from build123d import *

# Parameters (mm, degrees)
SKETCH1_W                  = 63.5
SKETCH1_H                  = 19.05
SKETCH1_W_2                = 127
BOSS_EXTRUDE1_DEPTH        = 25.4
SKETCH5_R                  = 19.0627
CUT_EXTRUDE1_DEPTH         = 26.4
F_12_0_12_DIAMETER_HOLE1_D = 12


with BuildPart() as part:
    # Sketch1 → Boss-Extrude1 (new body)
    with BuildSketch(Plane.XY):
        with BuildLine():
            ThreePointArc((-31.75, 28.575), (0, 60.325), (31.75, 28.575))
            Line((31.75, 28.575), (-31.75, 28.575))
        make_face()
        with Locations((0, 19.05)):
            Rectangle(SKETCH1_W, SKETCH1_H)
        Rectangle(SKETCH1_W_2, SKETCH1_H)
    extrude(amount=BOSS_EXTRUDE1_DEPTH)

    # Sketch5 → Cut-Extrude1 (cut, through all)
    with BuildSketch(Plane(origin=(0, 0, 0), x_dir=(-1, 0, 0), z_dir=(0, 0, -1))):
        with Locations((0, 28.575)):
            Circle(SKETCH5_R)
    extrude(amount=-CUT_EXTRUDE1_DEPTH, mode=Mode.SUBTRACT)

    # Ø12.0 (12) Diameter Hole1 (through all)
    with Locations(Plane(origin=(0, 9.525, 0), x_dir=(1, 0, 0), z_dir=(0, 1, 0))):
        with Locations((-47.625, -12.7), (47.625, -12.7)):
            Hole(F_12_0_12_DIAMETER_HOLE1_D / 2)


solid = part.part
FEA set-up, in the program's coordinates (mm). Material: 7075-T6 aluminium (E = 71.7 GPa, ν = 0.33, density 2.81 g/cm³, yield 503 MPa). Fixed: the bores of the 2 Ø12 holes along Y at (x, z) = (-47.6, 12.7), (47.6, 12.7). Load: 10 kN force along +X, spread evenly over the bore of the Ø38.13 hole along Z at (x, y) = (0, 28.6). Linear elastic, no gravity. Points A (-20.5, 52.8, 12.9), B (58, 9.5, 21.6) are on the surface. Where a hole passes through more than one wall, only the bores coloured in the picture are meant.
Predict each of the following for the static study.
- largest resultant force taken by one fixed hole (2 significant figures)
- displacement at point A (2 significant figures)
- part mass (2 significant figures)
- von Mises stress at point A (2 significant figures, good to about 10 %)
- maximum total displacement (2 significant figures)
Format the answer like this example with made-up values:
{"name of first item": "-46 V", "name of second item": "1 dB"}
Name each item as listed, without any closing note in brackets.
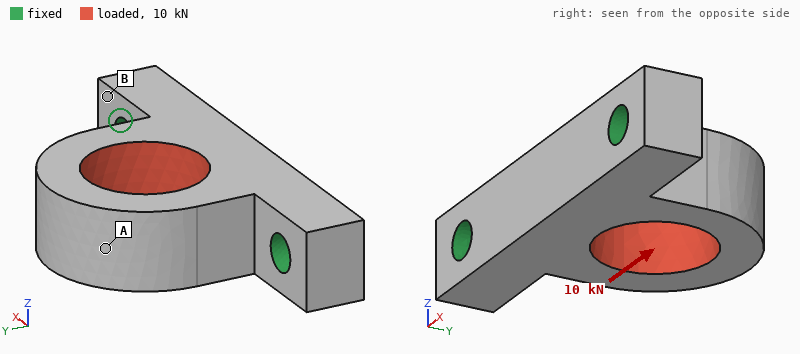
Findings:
{"largest resultant force taken by one fixed hole": "6.2 kN", "displacement at point A": "53 µm", "part mass": "280 g", "von Mises stress at point A": "20 MPa", "maximum total displacement": "54 µm"}
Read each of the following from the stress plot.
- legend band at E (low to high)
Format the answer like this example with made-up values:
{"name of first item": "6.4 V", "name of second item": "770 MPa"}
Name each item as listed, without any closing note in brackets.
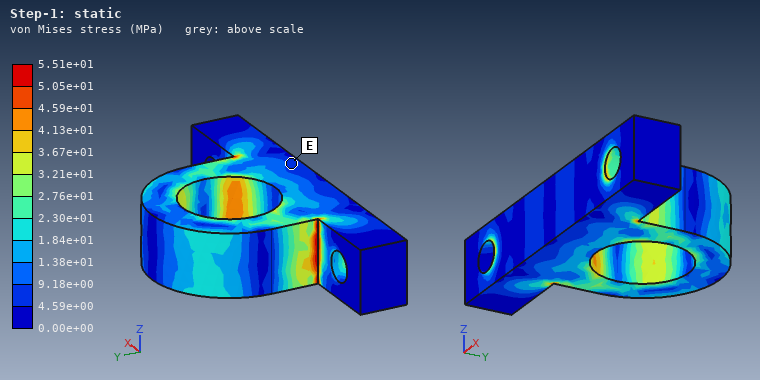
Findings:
{"legend band at E": "4.59e+00 to 9.18e+00 MPa"}
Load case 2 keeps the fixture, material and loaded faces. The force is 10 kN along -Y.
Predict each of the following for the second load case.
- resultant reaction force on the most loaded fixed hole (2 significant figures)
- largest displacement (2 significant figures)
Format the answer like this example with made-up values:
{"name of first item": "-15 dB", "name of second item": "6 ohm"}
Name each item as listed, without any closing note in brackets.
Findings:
{"resultant reaction force on the most loaded fixed hole": "5.2 kN", "largest displacement": "21 µm"}
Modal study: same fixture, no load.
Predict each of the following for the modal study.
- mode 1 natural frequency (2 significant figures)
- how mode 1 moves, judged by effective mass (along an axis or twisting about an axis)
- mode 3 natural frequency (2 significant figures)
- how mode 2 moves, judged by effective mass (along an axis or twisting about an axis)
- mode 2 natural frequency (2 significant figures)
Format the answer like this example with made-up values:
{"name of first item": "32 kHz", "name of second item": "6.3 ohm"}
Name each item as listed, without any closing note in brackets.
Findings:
{"mode 1 natural frequency": "3100 Hz", "how mode 1 moves, judged by effective mass": "along Z", "mode 3 natural frequency": "8300 Hz", "how mode 2 moves, judged by effective mass": "along X", "mode 2 natural frequency": "6300 Hz"}
